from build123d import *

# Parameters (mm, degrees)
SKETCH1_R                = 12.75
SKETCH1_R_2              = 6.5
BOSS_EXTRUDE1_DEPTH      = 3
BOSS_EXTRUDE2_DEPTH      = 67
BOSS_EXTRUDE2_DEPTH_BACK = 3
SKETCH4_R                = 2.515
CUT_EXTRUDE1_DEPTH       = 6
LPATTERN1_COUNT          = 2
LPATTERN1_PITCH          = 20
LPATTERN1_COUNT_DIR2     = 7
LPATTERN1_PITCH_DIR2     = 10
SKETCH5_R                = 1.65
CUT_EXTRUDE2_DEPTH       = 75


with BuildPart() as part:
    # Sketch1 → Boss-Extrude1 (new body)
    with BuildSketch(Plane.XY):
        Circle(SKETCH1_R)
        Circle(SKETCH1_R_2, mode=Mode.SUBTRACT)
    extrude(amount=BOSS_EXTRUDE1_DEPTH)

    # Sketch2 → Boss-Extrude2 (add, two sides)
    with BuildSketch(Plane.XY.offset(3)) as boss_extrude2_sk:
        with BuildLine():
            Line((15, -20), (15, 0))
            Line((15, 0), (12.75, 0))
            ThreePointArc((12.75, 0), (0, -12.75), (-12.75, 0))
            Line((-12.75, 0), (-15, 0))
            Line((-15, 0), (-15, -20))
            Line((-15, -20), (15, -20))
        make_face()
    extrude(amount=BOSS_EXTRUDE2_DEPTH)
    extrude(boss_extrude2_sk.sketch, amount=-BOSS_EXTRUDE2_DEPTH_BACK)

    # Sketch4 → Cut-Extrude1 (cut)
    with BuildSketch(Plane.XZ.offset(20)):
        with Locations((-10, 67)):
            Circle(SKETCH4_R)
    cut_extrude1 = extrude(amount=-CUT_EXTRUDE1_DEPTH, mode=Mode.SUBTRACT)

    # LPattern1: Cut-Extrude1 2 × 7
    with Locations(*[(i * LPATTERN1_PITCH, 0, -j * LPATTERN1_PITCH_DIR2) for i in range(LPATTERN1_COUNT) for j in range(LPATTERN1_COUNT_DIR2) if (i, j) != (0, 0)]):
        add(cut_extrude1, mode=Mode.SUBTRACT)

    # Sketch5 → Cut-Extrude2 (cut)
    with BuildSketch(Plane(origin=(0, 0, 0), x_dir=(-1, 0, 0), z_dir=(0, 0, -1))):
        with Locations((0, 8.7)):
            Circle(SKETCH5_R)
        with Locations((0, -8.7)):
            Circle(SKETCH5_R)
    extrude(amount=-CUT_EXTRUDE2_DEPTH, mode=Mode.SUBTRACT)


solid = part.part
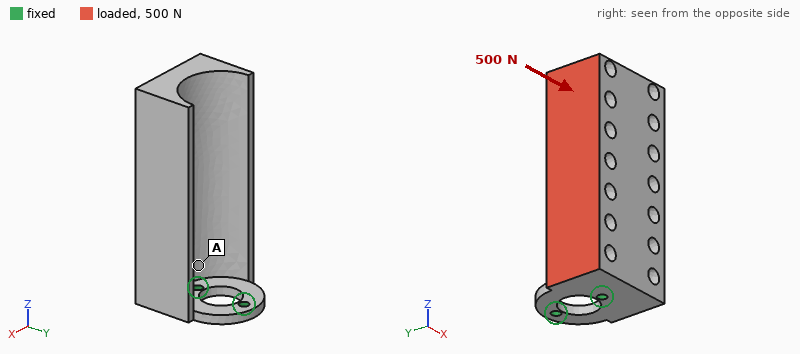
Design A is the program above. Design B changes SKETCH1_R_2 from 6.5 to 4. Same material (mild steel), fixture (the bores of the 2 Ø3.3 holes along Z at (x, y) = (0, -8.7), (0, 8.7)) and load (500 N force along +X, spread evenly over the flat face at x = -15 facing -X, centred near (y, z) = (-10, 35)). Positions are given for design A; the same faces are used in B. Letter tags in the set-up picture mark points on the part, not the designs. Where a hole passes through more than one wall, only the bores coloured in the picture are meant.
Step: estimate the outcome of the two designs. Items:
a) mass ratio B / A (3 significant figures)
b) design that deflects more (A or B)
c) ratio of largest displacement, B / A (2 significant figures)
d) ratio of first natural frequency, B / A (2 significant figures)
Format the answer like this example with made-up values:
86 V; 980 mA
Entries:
1.01; A; 0.88; 1.1
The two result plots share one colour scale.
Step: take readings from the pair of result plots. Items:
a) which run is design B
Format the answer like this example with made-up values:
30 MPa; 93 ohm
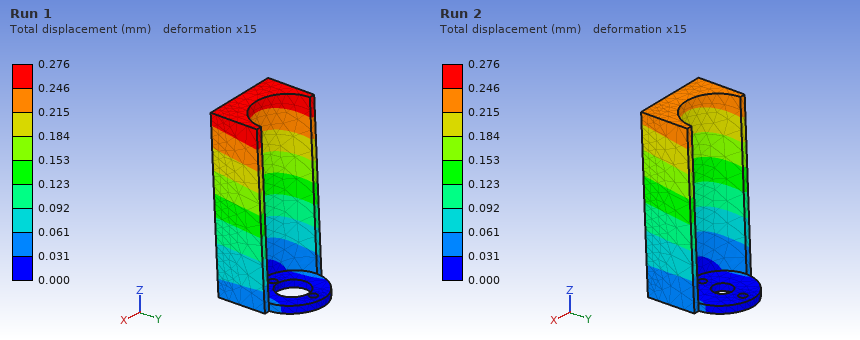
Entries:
Run 2
